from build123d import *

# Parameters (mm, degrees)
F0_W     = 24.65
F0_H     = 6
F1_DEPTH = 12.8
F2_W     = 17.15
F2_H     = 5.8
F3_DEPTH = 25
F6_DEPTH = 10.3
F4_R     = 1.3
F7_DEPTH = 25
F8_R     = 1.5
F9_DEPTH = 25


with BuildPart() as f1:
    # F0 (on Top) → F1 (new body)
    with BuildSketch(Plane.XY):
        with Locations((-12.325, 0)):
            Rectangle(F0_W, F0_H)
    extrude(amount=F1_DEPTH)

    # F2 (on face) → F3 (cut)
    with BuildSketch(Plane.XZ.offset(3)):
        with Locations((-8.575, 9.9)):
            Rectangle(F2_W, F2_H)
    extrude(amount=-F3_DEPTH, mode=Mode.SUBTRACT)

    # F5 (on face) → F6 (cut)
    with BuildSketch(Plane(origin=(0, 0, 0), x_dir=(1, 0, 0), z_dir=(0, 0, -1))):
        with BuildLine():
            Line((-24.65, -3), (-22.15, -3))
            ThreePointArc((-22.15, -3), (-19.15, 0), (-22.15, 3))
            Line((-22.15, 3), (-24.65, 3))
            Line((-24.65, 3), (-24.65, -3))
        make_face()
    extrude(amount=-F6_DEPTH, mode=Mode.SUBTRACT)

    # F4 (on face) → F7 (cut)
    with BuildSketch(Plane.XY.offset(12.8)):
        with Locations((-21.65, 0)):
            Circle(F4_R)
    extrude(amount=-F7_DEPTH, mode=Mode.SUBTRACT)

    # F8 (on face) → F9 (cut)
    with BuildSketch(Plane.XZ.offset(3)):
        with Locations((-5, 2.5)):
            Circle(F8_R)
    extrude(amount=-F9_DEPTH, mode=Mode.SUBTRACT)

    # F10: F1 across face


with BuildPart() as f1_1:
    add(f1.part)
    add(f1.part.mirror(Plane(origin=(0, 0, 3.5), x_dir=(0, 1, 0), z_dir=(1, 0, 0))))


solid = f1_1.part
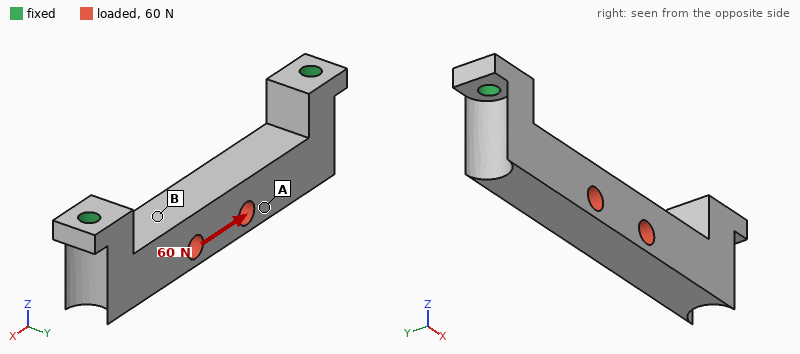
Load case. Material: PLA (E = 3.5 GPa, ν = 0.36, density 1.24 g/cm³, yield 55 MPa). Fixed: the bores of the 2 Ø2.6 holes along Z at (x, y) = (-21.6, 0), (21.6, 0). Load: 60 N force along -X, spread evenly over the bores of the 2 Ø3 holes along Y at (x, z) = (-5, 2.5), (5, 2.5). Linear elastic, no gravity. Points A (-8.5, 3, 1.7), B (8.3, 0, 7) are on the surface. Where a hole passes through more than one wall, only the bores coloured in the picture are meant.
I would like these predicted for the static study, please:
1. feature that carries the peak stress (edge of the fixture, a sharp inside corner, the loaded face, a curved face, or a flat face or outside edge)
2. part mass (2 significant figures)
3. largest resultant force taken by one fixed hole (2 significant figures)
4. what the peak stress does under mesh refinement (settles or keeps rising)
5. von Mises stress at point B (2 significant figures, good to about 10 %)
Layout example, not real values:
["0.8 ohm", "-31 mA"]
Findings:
["a sharp inside corner", "2.3 g", "32 N", "keeps rising", "2.1 MPa"]
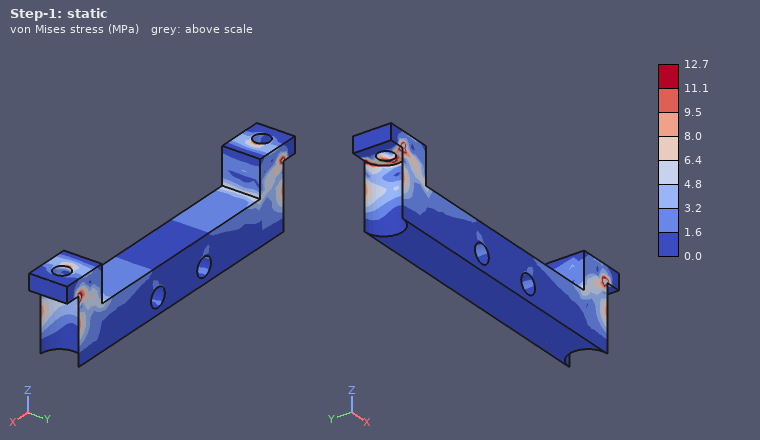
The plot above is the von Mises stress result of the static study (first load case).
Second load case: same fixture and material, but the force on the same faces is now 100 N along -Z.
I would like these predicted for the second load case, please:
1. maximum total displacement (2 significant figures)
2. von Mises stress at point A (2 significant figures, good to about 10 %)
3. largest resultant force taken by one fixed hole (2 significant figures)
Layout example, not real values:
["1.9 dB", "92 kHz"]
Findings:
["0.12 mm", "5.0 MPa", "68 N"]
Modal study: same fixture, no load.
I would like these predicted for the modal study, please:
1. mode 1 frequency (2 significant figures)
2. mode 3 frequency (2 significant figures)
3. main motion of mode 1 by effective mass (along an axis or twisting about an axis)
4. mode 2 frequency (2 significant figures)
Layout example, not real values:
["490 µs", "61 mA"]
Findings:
["2200 Hz", "4700 Hz", "along Y", "4500 Hz"]
